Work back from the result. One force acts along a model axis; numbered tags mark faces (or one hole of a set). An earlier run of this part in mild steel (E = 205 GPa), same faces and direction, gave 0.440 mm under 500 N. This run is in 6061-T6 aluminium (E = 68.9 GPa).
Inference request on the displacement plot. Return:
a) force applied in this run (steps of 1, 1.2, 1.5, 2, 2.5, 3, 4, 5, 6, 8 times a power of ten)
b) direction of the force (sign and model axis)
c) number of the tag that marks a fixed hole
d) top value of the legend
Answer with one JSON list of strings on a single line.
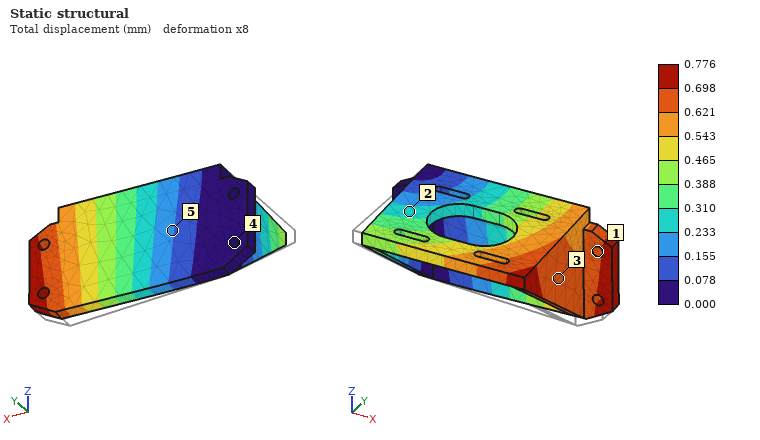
["300 N", "+Y", "4", "0.776 mm"]
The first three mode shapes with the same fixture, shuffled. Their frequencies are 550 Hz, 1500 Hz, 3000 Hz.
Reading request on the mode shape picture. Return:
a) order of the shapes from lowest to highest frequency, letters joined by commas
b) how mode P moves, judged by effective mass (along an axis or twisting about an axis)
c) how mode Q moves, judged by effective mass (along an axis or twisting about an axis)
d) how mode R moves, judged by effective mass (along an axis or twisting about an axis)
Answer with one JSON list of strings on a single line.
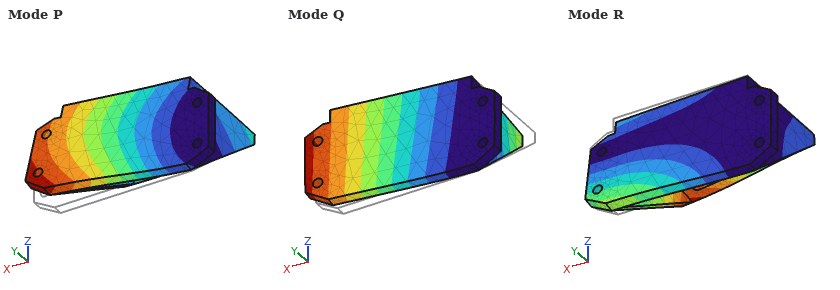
["Q, R, P", "along Z", "along Y", "along Z"]
